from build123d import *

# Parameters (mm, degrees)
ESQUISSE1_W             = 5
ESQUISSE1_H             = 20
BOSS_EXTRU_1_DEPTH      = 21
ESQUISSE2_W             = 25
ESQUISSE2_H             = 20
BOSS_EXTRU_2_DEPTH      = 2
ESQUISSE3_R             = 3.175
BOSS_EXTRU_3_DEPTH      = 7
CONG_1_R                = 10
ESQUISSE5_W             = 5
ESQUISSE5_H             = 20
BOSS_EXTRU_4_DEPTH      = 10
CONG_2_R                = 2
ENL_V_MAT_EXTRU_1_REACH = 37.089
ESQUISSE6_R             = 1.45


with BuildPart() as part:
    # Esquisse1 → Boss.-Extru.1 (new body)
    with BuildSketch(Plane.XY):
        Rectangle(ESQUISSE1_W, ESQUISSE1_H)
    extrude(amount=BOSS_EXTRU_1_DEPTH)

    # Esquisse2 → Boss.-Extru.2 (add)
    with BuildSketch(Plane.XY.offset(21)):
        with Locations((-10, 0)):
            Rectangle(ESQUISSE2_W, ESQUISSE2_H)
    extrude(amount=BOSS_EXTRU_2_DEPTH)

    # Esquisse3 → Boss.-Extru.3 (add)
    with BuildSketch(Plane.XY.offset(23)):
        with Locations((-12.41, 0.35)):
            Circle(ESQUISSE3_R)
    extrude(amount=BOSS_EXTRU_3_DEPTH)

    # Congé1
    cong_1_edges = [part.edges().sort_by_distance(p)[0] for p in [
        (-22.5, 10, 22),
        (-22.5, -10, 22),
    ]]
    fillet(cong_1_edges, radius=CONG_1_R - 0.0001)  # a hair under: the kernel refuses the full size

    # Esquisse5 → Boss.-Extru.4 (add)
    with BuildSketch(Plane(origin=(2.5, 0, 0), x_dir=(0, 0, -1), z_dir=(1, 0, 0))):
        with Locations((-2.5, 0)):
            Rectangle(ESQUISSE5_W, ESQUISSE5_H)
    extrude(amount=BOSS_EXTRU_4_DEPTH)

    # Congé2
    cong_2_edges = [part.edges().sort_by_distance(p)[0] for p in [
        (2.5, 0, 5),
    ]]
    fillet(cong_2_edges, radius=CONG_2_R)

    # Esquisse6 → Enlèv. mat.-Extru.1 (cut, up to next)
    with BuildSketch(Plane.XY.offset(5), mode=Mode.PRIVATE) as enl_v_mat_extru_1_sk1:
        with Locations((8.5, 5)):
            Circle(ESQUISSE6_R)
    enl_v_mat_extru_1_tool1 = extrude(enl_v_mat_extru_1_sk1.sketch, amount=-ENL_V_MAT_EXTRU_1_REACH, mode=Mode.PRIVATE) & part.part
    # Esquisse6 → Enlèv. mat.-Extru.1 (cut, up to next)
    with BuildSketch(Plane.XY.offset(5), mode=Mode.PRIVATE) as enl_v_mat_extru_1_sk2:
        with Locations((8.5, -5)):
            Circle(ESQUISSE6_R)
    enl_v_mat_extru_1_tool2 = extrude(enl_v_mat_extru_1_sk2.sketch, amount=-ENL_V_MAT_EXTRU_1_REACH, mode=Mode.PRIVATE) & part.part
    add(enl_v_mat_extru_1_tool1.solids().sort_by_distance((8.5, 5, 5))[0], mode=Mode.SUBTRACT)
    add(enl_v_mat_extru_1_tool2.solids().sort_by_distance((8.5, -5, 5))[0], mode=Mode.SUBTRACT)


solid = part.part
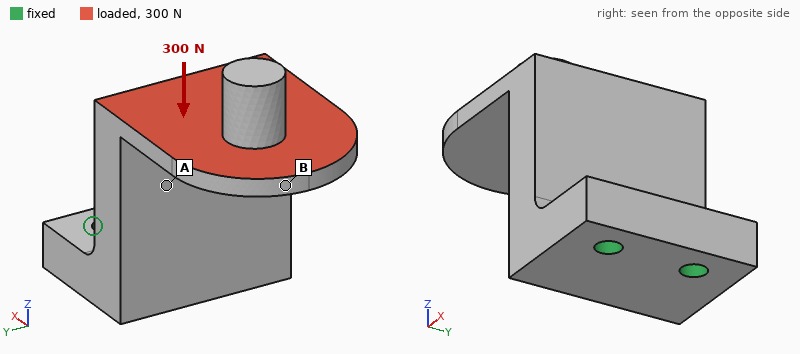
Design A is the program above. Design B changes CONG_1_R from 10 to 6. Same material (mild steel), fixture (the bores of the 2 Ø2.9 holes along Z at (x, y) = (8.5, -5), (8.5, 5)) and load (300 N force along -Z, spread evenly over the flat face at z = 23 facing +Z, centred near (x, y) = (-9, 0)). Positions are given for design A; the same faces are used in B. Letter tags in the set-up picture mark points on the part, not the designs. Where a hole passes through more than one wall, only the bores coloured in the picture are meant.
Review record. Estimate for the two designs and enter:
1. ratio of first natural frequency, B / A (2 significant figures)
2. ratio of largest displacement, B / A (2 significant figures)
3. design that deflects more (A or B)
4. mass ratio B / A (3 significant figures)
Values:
0.94
1.1
B
1.01
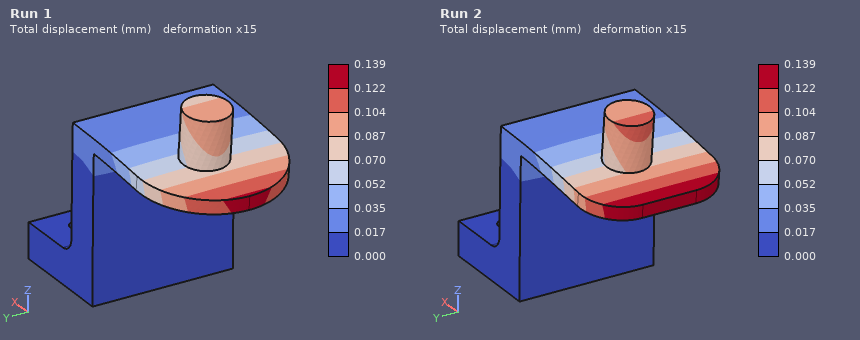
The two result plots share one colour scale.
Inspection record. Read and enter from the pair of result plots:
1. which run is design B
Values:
Run 2
